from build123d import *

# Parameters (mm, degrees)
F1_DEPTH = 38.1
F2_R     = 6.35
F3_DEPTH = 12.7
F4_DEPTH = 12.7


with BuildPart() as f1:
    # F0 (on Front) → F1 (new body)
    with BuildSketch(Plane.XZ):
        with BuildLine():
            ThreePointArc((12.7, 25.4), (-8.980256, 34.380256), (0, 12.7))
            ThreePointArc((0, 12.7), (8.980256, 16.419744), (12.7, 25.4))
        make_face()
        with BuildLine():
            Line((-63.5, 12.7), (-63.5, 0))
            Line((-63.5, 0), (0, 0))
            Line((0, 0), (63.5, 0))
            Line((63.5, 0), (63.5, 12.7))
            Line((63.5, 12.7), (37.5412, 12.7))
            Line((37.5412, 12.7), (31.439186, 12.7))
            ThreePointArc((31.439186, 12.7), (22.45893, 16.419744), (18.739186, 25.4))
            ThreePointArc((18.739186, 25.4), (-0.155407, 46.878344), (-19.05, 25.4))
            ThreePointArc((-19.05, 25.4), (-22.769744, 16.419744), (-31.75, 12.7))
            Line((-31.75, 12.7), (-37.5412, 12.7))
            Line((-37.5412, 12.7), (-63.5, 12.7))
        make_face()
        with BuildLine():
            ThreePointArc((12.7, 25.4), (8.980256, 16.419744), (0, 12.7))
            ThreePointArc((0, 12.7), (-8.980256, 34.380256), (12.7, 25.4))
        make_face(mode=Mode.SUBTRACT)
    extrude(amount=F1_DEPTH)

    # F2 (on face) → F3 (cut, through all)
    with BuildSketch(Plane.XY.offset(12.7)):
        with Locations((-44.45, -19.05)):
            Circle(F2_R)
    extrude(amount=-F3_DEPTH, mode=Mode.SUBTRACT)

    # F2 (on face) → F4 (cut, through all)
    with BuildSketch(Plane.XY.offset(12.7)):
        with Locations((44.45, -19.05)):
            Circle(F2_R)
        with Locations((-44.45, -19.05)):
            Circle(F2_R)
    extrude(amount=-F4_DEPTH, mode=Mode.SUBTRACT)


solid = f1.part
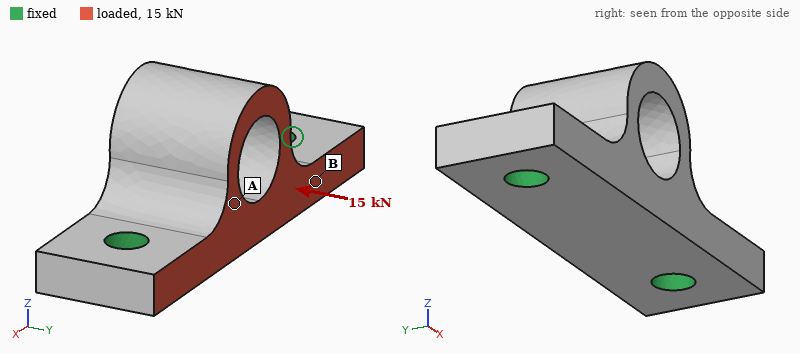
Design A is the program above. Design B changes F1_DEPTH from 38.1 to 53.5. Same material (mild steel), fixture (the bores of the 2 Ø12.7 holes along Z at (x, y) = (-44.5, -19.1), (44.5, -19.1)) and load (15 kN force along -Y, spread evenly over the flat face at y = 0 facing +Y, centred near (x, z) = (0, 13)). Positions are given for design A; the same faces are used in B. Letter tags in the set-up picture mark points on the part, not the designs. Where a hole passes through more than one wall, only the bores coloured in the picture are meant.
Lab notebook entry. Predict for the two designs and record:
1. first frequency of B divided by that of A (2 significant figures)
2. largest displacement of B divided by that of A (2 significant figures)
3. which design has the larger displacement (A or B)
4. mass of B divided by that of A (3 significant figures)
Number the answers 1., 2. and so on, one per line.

1. 0.83
2. 0.77
3. A
4. 1.42
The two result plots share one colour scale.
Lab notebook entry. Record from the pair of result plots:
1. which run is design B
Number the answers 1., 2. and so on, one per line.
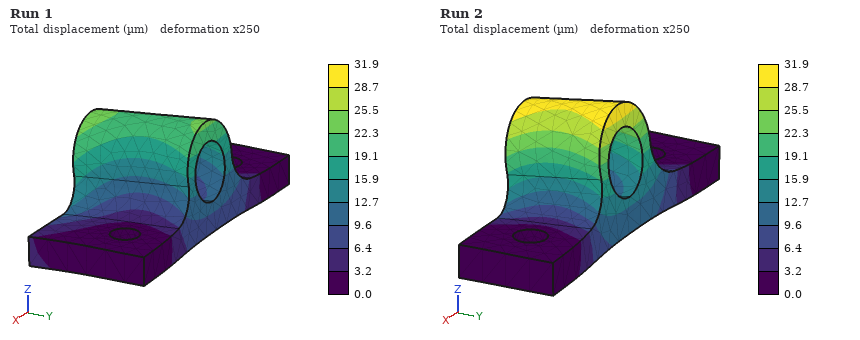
1. Run 1
